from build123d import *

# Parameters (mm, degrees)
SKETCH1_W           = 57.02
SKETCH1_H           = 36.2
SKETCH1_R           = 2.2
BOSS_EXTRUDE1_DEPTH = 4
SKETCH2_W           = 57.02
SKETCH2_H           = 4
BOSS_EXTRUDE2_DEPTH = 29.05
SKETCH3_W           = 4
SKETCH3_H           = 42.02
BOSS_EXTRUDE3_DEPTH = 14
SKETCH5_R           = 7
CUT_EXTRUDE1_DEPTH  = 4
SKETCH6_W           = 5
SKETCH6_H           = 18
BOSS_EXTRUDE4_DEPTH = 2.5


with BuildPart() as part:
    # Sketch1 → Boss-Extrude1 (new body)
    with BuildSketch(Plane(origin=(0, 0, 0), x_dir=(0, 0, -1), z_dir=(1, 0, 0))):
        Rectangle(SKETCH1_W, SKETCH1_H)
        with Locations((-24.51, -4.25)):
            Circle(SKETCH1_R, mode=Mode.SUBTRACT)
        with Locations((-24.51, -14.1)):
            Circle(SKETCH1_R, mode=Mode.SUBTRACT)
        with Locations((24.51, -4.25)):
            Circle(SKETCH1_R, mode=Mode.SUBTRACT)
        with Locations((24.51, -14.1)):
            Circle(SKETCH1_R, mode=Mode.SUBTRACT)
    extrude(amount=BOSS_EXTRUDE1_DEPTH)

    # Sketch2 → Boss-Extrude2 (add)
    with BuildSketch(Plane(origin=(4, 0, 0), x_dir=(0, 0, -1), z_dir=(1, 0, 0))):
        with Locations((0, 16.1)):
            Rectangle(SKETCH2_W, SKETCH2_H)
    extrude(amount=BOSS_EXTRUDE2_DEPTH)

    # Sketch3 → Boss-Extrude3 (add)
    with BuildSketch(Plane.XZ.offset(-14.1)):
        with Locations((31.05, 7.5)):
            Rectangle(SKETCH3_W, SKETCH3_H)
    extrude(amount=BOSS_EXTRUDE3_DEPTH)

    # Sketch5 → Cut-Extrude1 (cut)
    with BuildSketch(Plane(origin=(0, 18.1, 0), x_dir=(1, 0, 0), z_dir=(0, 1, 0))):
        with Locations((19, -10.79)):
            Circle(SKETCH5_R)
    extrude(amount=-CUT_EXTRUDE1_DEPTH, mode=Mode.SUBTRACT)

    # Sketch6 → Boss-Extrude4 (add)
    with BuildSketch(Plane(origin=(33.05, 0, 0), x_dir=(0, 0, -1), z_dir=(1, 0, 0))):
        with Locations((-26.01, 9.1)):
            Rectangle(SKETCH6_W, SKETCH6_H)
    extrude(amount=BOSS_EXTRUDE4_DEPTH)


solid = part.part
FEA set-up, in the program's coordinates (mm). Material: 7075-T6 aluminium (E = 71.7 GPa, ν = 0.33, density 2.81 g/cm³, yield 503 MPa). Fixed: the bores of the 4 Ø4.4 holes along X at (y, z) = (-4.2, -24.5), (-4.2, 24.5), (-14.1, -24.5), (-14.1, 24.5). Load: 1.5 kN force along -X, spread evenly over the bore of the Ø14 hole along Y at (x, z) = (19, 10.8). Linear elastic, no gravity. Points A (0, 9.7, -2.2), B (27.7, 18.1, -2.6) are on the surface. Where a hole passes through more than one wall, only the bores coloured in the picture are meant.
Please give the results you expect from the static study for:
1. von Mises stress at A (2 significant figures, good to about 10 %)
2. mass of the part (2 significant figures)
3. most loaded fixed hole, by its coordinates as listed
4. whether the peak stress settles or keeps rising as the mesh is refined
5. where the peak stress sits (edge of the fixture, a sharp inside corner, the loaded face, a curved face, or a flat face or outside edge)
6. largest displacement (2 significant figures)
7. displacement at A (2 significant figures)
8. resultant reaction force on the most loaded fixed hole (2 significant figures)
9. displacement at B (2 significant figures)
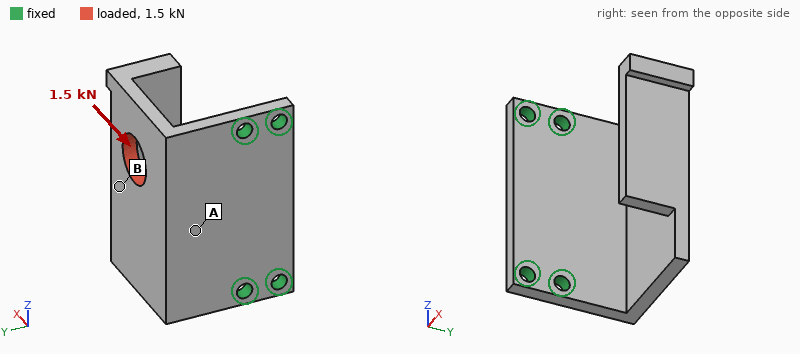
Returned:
61 MPa
47 g
(-4.2, 24.5)
keeps rising
edge of the fixture
0.71 mm
0.16 mm
1.6 kN
0.50 mm
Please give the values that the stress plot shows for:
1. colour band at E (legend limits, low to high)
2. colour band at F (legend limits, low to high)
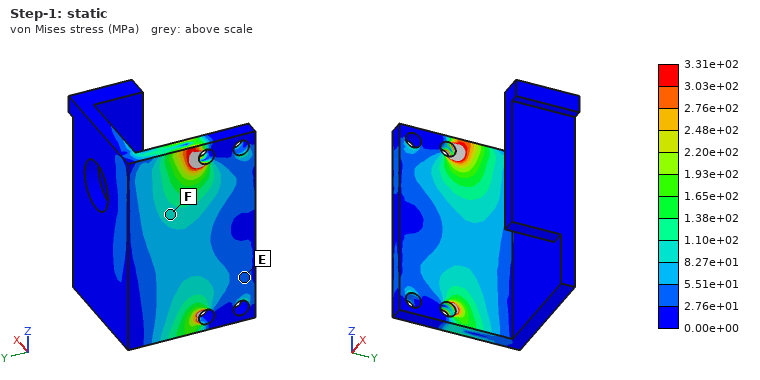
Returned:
2.76e+01 to 5.51e+01 MPa
8.27e+01 to 1.10e+02 MPa
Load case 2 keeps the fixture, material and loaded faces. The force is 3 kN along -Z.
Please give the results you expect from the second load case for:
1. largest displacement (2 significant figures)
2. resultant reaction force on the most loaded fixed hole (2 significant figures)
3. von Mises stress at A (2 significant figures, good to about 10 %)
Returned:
0.49 mm
2.1 kN
58 MPa
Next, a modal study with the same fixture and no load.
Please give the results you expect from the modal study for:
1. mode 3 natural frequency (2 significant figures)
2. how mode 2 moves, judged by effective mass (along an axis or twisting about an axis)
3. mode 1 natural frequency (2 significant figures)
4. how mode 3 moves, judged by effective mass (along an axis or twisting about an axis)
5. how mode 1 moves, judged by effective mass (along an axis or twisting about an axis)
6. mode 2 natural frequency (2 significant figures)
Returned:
2900 Hz
along Z
1200 Hz
along X
along Y
2200 Hz
